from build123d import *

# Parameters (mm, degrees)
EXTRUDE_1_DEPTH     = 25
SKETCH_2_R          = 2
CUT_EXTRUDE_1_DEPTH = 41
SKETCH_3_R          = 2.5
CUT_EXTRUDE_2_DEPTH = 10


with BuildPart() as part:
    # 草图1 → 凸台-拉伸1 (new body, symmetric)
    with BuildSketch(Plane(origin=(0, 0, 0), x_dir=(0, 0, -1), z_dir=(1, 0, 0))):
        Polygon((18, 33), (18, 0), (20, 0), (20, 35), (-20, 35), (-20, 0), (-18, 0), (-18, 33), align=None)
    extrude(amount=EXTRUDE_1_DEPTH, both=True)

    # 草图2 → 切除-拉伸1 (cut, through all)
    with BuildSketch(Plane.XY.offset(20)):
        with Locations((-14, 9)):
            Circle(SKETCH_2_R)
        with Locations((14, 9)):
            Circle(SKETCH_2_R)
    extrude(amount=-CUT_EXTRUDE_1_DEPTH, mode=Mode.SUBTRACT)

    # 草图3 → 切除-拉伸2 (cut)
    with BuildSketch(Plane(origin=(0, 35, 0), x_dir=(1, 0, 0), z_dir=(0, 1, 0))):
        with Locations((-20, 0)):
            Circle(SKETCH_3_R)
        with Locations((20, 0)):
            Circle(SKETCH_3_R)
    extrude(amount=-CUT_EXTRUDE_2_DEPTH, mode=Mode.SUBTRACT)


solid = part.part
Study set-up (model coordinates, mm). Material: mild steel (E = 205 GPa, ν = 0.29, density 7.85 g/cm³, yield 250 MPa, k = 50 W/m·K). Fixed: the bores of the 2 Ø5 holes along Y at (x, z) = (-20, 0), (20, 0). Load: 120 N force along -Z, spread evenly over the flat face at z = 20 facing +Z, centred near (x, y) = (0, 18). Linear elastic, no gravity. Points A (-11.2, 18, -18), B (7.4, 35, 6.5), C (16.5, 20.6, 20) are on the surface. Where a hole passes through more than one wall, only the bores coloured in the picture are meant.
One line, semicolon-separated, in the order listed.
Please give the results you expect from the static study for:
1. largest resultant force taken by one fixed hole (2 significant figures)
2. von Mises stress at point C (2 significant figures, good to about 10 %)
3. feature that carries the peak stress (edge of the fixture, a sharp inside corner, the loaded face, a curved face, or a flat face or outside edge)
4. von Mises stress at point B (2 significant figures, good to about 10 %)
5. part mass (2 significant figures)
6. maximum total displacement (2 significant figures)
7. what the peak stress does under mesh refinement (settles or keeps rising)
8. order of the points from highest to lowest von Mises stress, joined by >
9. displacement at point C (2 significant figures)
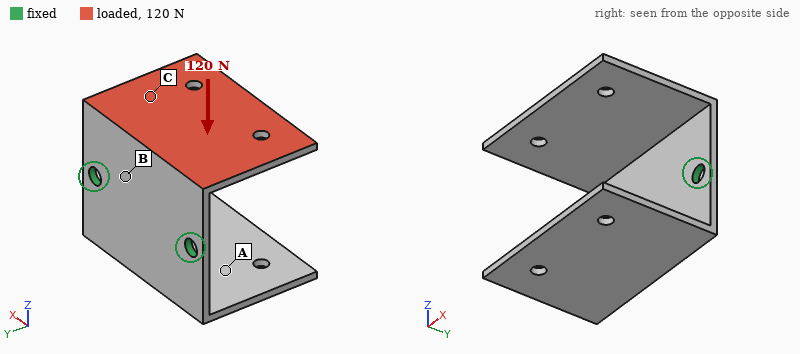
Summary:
61 N; 20 MPa; edge of the fixture; 43 MPa; 82 g; 0.25 mm; keeps rising; B > C > A; 0.10 mm
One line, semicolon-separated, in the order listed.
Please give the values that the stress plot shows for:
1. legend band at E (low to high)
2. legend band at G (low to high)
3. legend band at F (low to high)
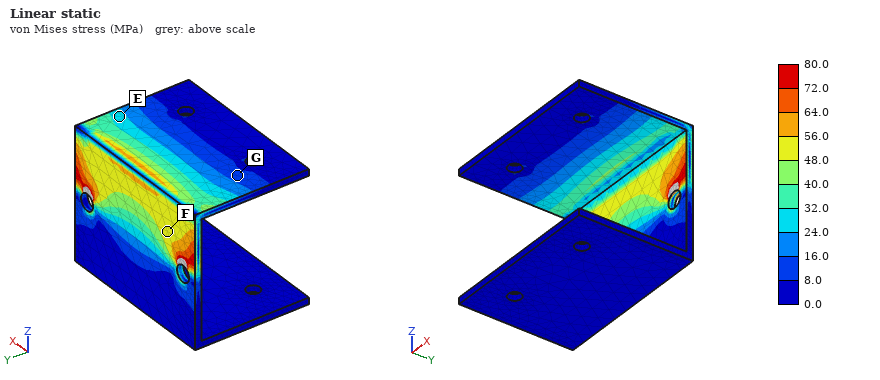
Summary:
24.0 to 32.0 MPa; 8.0 to 16.0 MPa; 48.0 to 56.0 MPa
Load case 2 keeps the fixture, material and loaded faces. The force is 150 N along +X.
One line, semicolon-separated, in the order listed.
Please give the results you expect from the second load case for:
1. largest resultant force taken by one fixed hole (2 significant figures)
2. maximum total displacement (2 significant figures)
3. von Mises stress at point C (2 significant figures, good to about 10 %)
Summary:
120 N; 50 µm; 6.1 MPa
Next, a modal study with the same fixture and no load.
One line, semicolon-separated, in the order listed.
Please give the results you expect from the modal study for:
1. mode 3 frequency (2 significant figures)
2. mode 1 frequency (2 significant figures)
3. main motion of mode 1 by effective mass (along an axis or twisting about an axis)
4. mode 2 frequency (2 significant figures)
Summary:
1700 Hz; 750 Hz; along Z; 800 Hz
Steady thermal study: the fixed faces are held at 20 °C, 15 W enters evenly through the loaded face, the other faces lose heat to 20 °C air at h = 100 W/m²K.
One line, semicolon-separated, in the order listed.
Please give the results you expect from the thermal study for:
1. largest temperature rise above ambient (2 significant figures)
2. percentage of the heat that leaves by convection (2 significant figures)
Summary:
45 K; 72 %
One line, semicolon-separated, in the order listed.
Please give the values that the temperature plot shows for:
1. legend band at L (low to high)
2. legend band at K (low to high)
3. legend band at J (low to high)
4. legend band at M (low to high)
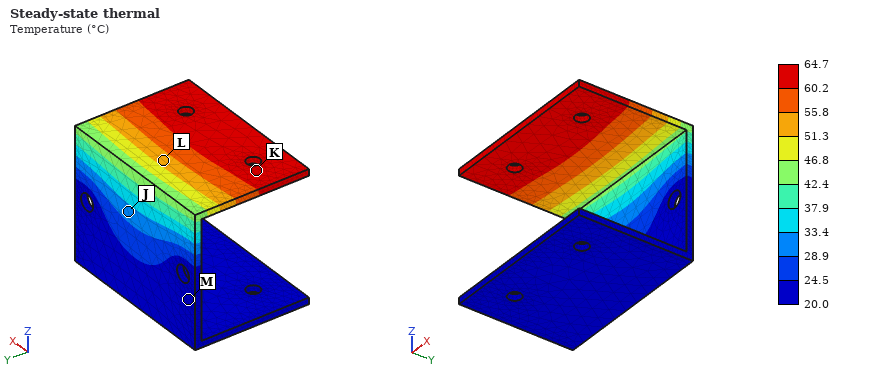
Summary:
51.3 to 55.8 °C; 60.2 to 64.7 °C; 28.9 to 33.4 °C; 20.0 to 24.5 °C
